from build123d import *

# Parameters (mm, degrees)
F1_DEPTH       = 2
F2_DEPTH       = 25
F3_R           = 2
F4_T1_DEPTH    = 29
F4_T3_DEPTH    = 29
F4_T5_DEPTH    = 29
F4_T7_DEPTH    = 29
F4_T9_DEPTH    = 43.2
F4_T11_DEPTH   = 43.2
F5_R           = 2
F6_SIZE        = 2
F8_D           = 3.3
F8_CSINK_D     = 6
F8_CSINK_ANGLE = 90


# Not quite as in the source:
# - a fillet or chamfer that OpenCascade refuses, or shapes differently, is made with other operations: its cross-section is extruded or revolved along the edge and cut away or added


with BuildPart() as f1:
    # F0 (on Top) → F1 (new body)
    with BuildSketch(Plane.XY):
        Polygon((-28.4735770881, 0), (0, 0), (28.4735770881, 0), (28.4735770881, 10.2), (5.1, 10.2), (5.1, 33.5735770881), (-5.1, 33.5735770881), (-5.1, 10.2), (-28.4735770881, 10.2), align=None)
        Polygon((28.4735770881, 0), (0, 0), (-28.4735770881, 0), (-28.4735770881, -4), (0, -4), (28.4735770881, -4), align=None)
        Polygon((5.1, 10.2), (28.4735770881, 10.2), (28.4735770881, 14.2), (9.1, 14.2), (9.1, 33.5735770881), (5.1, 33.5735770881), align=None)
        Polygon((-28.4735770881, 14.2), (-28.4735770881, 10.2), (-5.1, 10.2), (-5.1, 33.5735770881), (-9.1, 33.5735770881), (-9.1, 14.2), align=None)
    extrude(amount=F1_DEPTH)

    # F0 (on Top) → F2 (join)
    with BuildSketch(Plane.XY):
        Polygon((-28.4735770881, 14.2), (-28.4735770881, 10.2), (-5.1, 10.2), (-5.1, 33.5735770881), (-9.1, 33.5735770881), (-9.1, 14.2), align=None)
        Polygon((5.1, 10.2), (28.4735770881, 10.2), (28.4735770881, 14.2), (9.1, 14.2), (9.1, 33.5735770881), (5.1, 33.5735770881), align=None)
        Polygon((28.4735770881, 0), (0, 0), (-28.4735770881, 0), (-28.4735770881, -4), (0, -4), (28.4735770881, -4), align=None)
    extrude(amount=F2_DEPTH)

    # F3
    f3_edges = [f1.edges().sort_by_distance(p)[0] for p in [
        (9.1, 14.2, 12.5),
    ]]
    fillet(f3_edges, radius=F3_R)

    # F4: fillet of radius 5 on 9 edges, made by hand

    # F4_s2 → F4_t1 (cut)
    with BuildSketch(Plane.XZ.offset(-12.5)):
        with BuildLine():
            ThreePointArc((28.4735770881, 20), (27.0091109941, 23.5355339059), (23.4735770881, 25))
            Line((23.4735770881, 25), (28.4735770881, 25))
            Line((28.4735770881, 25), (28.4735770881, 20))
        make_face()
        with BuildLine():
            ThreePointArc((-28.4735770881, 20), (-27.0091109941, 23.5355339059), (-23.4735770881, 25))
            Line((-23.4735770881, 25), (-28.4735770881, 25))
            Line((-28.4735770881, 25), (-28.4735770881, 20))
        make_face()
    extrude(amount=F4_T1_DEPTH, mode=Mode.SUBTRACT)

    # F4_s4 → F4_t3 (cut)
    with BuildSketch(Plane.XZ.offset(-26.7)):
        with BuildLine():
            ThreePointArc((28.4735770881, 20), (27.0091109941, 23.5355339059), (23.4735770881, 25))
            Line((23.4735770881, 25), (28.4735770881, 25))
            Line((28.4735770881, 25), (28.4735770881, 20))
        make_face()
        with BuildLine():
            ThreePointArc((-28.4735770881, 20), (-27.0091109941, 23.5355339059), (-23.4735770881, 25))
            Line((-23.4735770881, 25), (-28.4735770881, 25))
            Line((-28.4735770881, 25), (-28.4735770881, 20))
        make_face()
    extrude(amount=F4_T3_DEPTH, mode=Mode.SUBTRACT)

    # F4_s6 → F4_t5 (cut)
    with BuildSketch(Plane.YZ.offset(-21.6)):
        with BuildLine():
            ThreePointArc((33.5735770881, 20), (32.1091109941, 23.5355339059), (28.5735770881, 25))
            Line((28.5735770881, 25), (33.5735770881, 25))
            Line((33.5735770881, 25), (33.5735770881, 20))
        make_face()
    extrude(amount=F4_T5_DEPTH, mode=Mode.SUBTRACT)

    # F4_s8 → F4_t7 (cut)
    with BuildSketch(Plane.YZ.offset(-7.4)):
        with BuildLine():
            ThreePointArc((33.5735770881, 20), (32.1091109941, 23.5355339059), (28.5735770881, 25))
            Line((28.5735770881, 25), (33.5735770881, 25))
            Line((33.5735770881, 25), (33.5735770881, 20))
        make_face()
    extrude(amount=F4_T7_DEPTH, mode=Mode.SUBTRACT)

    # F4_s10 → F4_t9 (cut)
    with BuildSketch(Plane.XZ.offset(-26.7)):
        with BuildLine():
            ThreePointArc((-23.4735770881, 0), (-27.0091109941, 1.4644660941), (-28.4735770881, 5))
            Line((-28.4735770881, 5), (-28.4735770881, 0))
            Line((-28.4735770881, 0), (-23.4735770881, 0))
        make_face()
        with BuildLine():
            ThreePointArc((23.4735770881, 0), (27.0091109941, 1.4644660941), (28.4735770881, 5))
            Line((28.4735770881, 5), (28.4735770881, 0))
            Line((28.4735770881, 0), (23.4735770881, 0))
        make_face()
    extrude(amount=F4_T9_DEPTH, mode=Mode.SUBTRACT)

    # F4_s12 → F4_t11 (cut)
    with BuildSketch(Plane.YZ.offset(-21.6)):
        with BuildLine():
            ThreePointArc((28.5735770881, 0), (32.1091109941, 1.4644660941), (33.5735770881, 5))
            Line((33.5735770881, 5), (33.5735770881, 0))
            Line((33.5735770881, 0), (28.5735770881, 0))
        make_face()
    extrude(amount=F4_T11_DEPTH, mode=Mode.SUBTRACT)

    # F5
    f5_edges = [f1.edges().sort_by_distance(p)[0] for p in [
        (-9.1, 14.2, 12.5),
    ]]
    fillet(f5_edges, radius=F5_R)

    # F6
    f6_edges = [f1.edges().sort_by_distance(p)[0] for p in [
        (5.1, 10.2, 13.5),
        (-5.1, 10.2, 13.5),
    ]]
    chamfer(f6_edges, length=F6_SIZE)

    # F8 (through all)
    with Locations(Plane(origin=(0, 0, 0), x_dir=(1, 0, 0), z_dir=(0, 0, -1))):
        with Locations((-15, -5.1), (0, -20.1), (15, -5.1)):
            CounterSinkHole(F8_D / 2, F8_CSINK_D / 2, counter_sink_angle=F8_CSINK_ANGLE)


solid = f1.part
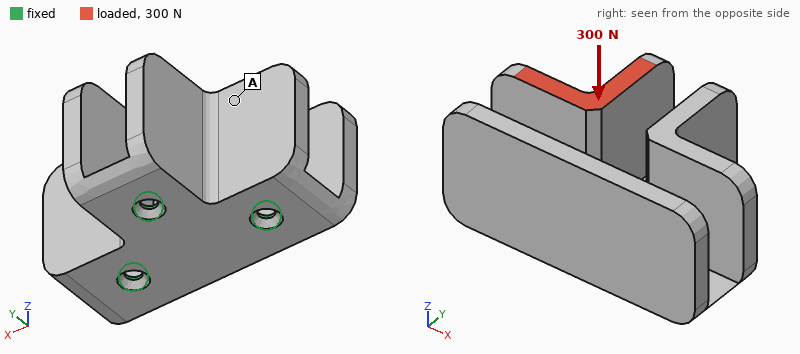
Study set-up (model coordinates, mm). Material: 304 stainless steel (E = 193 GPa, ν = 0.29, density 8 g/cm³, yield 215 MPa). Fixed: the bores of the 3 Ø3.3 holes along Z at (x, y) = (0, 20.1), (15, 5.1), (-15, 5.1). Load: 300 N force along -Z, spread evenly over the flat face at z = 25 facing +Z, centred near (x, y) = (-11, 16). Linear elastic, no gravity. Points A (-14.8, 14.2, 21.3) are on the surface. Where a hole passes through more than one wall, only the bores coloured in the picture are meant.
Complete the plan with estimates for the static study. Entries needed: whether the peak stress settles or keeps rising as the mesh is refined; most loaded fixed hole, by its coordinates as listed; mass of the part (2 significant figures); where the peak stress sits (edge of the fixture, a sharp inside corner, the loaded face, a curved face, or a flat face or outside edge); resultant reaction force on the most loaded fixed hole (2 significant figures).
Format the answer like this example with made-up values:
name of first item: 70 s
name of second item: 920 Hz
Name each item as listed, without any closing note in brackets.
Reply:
whether the peak stress settles or keeps rising as the mesh is refined: keeps rising
most loaded fixed hole, by its coordinates as listed: (0, 20.1)
mass of the part: 120 g
where the peak stress sits: edge of the fixture
resultant reaction force on the most loaded fixed hole: 190 N
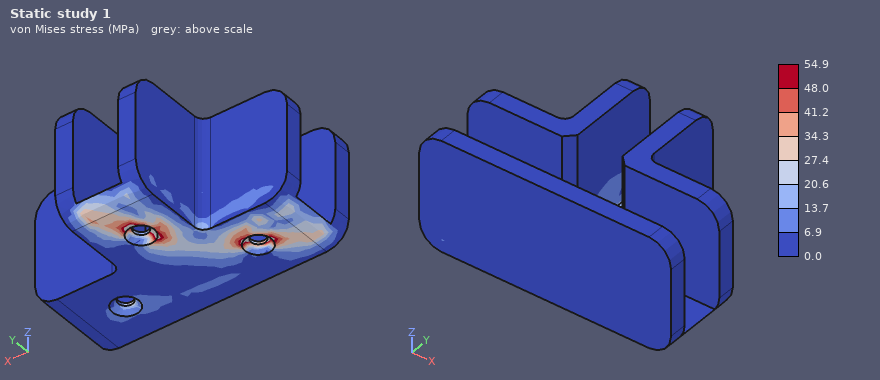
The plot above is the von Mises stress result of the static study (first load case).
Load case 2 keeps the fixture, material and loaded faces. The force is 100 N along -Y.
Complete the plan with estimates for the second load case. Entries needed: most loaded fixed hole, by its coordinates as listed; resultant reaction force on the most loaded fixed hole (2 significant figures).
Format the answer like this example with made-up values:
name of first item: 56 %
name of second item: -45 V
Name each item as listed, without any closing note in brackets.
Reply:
most loaded fixed hole, by its coordinates as listed: (0, 20.1)
resultant reaction force on the most loaded fixed hole: 170 N
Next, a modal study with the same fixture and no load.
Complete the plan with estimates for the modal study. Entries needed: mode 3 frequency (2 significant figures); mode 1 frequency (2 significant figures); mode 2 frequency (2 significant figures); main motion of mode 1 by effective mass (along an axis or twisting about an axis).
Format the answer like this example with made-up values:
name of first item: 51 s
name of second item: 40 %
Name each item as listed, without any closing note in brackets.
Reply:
mode 3 frequency: 2300 Hz
mode 1 frequency: 1400 Hz
mode 2 frequency: 2000 Hz
main motion of mode 1 by effective mass: along Y
